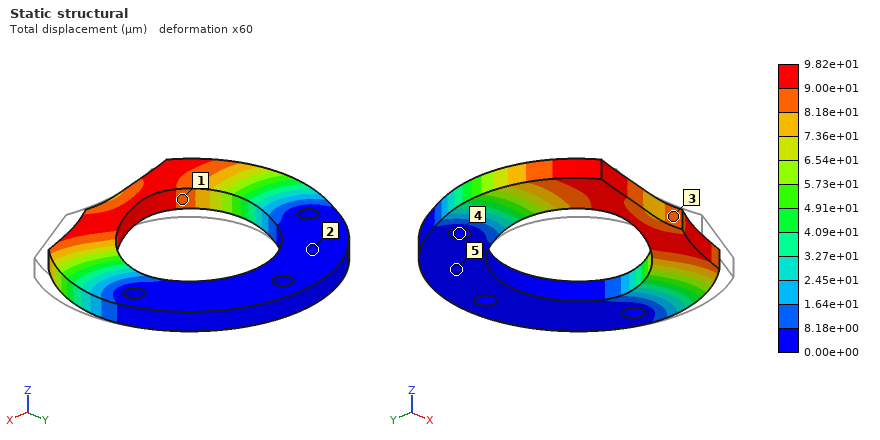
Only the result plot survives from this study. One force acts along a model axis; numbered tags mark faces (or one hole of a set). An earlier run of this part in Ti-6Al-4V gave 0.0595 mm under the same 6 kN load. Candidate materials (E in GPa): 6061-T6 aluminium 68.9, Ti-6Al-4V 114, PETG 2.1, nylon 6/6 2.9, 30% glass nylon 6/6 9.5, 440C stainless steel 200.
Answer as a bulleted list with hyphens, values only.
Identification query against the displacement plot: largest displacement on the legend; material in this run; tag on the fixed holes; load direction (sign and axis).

- 9.82e+01 µm
- 6061-T6 aluminium
- 4
- -X
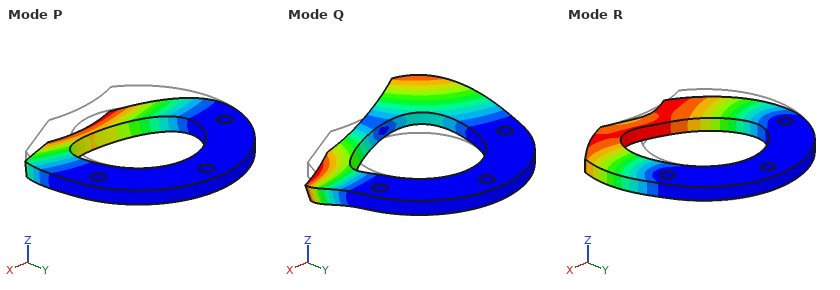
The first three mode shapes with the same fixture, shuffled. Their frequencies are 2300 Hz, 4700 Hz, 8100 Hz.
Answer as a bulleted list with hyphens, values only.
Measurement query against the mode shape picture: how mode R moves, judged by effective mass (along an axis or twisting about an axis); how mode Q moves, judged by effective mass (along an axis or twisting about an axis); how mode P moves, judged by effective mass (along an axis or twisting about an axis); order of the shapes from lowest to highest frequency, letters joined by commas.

- along X
- twisting about Y
- along Z
- P, Q, R
